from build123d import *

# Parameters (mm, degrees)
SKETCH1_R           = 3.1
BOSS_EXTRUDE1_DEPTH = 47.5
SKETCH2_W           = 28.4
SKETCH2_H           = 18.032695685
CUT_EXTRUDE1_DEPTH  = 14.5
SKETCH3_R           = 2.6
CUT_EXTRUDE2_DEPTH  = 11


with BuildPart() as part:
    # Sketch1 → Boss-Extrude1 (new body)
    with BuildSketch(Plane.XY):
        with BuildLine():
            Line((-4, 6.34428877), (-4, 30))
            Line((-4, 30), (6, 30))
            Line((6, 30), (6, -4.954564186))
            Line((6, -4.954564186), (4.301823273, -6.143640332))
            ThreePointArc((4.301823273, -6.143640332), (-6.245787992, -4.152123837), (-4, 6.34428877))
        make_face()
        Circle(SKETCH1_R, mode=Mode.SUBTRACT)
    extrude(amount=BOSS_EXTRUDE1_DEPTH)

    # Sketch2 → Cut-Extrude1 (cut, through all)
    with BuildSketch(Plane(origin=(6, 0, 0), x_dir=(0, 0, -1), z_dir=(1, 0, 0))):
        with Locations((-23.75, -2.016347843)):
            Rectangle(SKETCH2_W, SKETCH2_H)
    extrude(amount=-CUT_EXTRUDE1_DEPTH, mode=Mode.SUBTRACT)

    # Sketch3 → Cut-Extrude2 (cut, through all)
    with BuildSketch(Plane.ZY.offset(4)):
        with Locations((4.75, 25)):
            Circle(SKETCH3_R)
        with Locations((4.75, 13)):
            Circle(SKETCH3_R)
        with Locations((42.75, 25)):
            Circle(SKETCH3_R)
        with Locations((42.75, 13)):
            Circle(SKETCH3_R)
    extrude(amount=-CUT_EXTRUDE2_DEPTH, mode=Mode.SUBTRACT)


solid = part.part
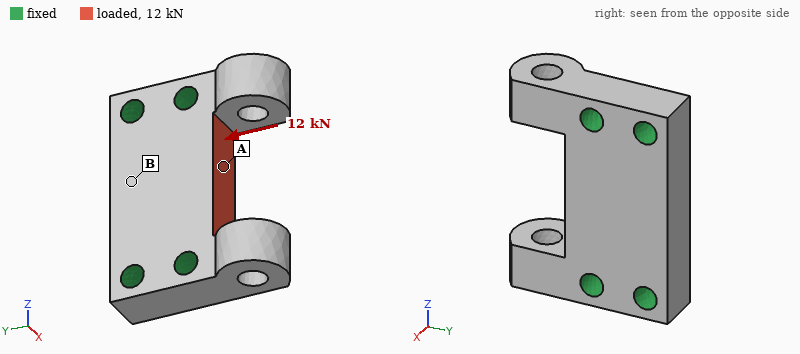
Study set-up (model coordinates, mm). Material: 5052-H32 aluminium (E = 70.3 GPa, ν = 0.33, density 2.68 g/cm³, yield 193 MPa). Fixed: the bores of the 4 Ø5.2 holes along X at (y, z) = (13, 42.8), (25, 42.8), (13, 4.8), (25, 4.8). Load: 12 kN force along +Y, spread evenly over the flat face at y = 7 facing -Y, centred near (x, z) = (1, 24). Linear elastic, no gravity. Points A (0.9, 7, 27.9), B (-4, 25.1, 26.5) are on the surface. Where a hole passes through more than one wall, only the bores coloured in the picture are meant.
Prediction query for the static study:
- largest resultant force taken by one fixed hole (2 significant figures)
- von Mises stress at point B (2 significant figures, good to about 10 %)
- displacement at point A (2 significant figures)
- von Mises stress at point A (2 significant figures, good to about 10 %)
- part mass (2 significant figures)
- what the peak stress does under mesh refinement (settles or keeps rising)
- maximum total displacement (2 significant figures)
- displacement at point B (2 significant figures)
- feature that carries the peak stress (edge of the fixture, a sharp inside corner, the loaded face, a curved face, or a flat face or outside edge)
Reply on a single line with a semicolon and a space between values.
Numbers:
3.6 kN; 15 MPa; 18 µm; 47 MPa; 34 g; keeps rising; 19 µm; 12 µm; edge of the fixture
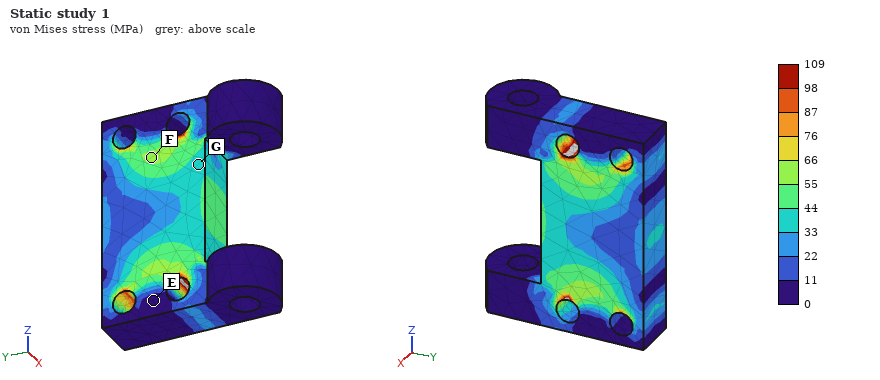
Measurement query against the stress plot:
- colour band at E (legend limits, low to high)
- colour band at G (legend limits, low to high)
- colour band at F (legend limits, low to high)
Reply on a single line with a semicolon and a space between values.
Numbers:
0 to 11 MPa; 33 to 44 MPa; 55 to 66 MPa
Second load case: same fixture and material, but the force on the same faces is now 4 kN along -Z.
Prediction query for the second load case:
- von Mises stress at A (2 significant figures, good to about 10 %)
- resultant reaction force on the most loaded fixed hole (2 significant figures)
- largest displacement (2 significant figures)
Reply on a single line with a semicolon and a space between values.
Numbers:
25 MPa; 1.7 kN; 4.4 µm
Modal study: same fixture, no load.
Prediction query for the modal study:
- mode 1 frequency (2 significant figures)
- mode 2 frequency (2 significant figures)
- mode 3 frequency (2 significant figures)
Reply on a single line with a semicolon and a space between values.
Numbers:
18 kHz; 18 kHz; 19 kHz
